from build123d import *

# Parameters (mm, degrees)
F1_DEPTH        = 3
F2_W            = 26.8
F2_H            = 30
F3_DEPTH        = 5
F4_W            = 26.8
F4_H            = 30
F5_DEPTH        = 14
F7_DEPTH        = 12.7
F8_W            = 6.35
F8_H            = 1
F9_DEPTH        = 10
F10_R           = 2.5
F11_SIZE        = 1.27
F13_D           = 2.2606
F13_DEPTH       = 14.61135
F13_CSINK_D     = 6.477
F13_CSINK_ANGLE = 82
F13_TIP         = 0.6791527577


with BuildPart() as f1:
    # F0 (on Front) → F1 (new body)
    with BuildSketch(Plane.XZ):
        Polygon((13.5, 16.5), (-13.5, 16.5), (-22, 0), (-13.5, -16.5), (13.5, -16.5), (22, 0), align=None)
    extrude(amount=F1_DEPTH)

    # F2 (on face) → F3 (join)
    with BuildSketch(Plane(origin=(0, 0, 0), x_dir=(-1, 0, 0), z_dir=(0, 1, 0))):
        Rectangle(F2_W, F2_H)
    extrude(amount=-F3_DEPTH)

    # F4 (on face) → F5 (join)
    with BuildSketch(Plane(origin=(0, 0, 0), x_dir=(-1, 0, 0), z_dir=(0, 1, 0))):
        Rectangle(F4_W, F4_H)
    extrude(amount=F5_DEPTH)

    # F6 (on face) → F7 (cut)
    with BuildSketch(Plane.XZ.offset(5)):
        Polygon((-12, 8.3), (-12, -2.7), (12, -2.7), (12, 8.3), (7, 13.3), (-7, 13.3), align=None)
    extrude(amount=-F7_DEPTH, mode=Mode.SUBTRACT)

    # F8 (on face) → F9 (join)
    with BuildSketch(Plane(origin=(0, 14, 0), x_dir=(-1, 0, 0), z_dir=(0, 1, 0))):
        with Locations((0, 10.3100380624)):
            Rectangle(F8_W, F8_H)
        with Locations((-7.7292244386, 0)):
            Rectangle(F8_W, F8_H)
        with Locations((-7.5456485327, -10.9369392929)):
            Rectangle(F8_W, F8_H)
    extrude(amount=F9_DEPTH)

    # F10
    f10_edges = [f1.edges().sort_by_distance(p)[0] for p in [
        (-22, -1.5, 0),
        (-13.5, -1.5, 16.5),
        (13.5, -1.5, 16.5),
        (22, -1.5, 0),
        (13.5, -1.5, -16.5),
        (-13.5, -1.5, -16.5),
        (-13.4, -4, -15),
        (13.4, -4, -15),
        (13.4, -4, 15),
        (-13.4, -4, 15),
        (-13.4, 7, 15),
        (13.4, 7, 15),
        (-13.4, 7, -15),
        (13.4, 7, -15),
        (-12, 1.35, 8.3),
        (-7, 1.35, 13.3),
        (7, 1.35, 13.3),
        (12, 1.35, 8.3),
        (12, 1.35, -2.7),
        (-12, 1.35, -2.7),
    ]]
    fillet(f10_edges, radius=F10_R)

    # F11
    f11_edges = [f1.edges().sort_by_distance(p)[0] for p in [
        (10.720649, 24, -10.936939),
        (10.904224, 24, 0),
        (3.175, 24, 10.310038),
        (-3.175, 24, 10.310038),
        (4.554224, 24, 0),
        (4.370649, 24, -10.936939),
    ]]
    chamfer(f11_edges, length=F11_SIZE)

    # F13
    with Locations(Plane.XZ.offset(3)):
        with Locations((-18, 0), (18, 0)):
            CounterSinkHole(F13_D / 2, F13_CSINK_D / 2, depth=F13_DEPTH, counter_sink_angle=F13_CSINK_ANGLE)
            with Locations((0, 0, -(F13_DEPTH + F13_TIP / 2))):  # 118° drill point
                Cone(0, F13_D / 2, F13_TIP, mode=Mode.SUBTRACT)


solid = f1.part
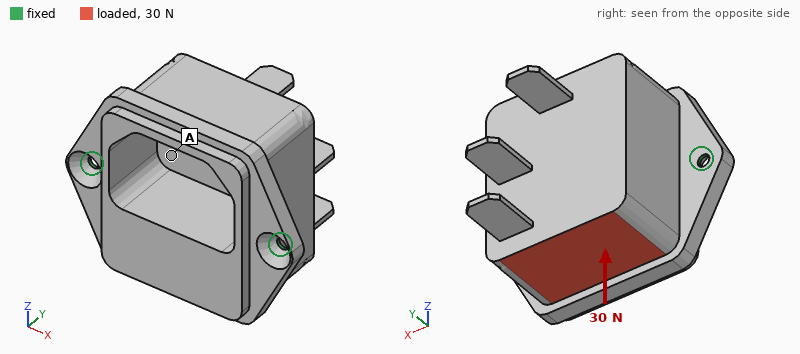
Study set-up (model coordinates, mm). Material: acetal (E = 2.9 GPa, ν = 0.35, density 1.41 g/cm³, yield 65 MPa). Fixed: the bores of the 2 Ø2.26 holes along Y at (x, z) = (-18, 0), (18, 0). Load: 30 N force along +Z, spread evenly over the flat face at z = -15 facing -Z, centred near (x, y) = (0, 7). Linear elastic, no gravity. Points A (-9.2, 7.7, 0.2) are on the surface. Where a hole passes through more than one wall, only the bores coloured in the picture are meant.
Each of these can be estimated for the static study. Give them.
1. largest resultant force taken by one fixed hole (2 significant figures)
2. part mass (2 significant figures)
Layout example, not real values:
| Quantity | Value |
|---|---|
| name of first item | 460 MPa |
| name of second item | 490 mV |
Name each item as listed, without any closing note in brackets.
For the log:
| Quantity | Value |
|---|---|
| largest resultant force taken by one fixed hole | 15 N |
| part mass | 17 g |
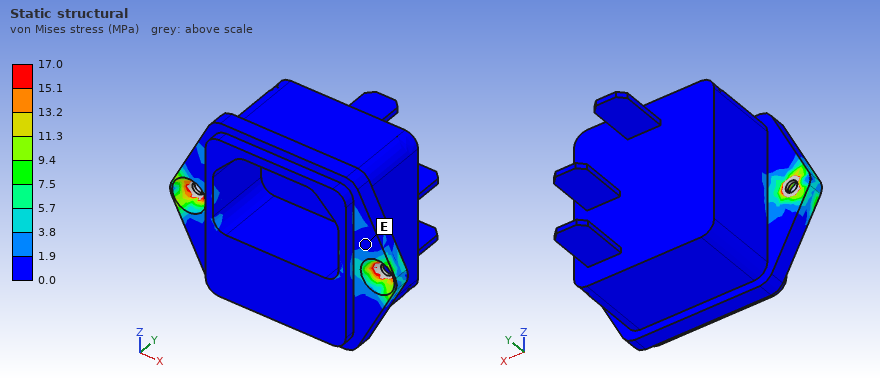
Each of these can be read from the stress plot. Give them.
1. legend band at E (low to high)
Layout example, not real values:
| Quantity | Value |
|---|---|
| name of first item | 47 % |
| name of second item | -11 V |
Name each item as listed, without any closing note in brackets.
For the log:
| Quantity | Value |
|---|---|
| legend band at E | 0.0 to 1.9 MPa |
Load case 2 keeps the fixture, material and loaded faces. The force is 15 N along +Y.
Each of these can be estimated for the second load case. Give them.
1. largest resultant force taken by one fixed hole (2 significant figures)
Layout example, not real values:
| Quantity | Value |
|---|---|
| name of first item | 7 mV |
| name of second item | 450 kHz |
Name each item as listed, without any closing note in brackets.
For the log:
| Quantity | Value |
|---|---|
| largest resultant force taken by one fixed hole | 7.8 N |
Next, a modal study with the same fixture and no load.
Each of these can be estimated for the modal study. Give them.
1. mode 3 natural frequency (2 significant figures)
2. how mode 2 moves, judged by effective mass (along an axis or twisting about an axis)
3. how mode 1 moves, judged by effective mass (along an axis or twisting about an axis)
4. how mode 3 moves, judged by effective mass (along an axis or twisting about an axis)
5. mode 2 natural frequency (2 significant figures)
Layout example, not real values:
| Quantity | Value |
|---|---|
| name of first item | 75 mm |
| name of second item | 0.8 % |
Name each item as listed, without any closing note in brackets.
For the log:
| Quantity | Value |
|---|---|
| mode 3 natural frequency | 1900 Hz |
| how mode 2 moves, judged by effective mass | along Y |
| how mode 1 moves, judged by effective mass | along Z |
| how mode 3 moves, judged by effective mass | along X |
| mode 2 natural frequency | 1700 Hz |
